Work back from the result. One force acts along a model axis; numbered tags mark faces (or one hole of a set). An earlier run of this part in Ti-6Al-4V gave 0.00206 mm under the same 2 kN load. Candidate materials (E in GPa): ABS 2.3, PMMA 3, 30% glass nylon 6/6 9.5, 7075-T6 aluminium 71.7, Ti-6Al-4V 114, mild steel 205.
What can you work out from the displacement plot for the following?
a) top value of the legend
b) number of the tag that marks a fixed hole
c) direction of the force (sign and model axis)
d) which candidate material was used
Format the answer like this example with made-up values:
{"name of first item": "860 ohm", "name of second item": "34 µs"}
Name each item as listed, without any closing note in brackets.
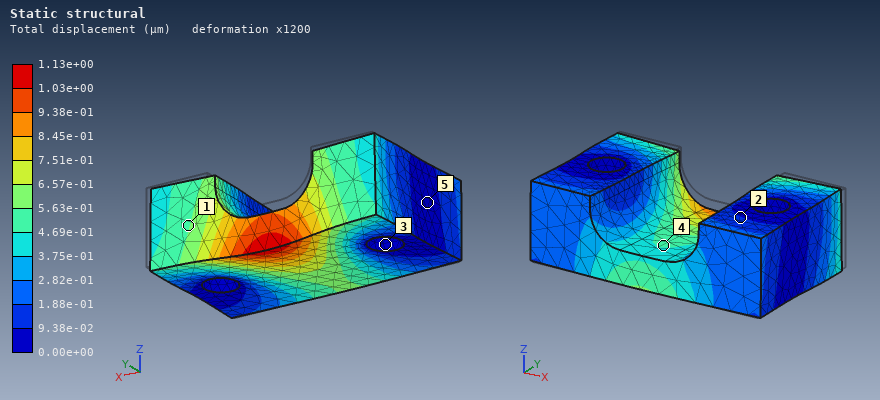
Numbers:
{"top value of the legend": "1.13e+00 µm", "number of the tag that marks a fixed hole": "3", "direction of the force": "-Y", "which candidate material was used": "mild steel"}
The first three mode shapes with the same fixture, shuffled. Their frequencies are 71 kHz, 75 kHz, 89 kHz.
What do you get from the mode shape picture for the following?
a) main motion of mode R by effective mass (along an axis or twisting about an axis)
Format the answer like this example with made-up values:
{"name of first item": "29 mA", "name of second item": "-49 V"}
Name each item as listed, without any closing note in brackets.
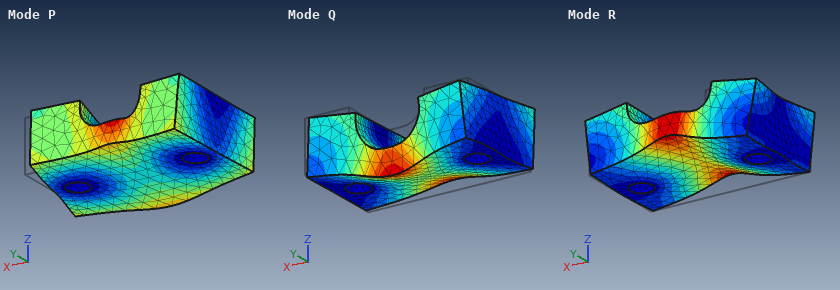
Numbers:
{"main motion of mode R by effective mass": "along Z"}
